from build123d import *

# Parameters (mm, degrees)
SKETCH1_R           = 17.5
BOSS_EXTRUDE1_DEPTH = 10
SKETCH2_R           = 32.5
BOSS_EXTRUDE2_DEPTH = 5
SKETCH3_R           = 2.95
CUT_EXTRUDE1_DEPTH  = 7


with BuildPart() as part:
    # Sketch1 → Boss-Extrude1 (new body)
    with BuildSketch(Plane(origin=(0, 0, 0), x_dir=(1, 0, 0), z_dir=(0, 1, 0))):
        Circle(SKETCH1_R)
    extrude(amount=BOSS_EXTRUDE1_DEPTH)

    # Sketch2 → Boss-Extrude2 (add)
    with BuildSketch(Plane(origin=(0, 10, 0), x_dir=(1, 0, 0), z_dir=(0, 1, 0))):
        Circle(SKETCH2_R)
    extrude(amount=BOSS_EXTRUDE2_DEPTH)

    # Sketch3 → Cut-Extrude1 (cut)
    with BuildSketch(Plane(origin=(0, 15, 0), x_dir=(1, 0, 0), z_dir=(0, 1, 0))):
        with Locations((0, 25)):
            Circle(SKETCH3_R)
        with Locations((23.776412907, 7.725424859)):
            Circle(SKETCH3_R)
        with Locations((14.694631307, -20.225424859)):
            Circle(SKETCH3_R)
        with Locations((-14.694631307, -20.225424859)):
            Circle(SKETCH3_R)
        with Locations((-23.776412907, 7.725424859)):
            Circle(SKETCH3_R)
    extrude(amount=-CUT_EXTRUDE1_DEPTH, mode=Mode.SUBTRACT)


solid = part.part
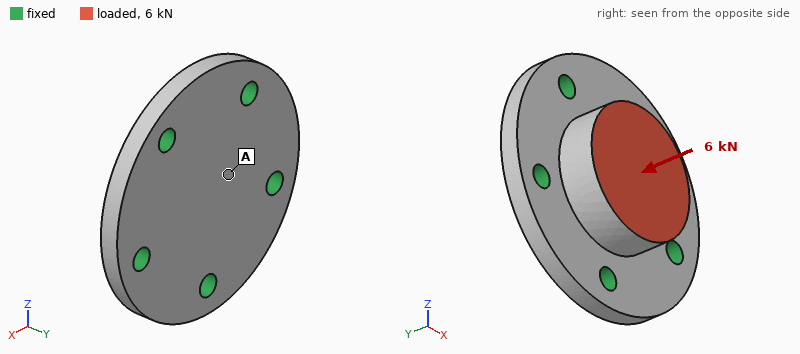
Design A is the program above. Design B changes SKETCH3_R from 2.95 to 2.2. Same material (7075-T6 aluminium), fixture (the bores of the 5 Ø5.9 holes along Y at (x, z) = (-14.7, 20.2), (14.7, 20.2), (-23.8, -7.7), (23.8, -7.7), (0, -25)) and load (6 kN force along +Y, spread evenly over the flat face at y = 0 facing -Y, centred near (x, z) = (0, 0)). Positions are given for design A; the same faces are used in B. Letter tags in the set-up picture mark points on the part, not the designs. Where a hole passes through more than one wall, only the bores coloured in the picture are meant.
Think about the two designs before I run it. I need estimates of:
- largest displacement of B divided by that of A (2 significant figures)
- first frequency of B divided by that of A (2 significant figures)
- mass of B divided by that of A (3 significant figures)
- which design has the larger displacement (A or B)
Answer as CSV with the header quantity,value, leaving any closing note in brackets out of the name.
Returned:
quantity,value
largest displacement of B divided by that of A,1.2
first frequency of B divided by that of A,0.90
mass of B divided by that of A,1.01
which design has the larger displacement,B
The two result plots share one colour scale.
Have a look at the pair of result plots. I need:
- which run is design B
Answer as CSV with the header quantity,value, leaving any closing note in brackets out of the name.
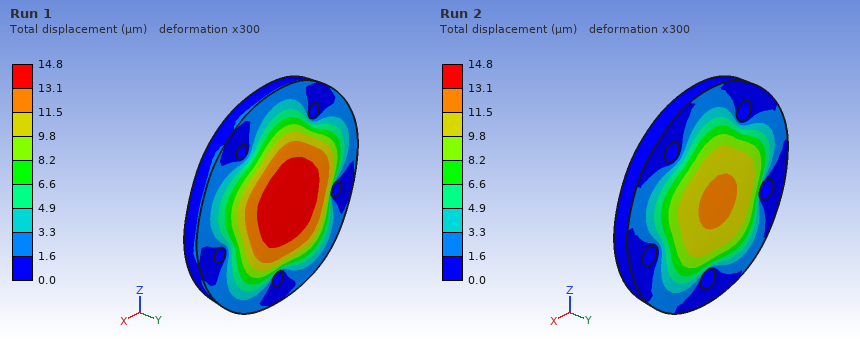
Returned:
quantity,value
which run is design B,Run 1
